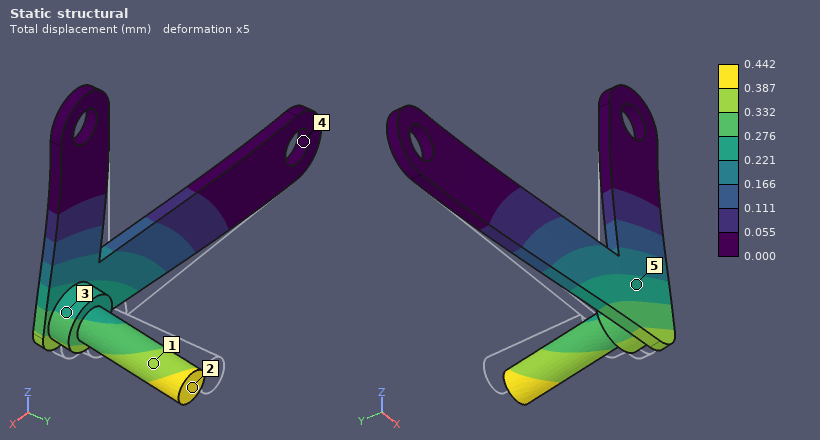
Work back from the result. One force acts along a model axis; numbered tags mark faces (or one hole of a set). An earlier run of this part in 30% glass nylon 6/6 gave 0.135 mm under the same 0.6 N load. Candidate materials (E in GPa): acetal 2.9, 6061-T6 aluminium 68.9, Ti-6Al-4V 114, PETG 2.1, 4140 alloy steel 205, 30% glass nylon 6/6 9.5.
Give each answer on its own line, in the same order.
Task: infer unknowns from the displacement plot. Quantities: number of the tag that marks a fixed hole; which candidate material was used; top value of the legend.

4
acetal
0.442 mm
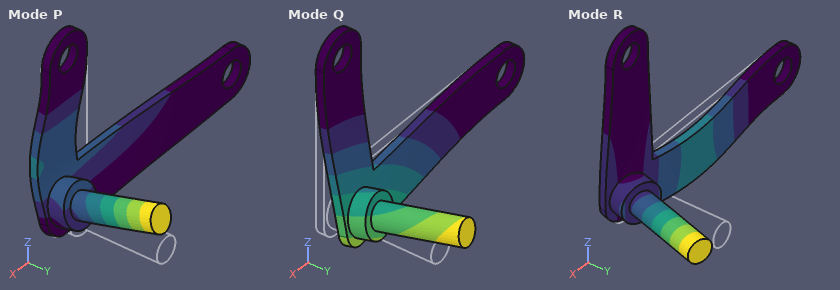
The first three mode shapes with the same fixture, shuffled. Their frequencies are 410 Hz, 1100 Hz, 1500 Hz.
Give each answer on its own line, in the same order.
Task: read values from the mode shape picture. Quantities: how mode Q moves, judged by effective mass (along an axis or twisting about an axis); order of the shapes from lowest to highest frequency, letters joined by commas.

along Y
Q, R, P
